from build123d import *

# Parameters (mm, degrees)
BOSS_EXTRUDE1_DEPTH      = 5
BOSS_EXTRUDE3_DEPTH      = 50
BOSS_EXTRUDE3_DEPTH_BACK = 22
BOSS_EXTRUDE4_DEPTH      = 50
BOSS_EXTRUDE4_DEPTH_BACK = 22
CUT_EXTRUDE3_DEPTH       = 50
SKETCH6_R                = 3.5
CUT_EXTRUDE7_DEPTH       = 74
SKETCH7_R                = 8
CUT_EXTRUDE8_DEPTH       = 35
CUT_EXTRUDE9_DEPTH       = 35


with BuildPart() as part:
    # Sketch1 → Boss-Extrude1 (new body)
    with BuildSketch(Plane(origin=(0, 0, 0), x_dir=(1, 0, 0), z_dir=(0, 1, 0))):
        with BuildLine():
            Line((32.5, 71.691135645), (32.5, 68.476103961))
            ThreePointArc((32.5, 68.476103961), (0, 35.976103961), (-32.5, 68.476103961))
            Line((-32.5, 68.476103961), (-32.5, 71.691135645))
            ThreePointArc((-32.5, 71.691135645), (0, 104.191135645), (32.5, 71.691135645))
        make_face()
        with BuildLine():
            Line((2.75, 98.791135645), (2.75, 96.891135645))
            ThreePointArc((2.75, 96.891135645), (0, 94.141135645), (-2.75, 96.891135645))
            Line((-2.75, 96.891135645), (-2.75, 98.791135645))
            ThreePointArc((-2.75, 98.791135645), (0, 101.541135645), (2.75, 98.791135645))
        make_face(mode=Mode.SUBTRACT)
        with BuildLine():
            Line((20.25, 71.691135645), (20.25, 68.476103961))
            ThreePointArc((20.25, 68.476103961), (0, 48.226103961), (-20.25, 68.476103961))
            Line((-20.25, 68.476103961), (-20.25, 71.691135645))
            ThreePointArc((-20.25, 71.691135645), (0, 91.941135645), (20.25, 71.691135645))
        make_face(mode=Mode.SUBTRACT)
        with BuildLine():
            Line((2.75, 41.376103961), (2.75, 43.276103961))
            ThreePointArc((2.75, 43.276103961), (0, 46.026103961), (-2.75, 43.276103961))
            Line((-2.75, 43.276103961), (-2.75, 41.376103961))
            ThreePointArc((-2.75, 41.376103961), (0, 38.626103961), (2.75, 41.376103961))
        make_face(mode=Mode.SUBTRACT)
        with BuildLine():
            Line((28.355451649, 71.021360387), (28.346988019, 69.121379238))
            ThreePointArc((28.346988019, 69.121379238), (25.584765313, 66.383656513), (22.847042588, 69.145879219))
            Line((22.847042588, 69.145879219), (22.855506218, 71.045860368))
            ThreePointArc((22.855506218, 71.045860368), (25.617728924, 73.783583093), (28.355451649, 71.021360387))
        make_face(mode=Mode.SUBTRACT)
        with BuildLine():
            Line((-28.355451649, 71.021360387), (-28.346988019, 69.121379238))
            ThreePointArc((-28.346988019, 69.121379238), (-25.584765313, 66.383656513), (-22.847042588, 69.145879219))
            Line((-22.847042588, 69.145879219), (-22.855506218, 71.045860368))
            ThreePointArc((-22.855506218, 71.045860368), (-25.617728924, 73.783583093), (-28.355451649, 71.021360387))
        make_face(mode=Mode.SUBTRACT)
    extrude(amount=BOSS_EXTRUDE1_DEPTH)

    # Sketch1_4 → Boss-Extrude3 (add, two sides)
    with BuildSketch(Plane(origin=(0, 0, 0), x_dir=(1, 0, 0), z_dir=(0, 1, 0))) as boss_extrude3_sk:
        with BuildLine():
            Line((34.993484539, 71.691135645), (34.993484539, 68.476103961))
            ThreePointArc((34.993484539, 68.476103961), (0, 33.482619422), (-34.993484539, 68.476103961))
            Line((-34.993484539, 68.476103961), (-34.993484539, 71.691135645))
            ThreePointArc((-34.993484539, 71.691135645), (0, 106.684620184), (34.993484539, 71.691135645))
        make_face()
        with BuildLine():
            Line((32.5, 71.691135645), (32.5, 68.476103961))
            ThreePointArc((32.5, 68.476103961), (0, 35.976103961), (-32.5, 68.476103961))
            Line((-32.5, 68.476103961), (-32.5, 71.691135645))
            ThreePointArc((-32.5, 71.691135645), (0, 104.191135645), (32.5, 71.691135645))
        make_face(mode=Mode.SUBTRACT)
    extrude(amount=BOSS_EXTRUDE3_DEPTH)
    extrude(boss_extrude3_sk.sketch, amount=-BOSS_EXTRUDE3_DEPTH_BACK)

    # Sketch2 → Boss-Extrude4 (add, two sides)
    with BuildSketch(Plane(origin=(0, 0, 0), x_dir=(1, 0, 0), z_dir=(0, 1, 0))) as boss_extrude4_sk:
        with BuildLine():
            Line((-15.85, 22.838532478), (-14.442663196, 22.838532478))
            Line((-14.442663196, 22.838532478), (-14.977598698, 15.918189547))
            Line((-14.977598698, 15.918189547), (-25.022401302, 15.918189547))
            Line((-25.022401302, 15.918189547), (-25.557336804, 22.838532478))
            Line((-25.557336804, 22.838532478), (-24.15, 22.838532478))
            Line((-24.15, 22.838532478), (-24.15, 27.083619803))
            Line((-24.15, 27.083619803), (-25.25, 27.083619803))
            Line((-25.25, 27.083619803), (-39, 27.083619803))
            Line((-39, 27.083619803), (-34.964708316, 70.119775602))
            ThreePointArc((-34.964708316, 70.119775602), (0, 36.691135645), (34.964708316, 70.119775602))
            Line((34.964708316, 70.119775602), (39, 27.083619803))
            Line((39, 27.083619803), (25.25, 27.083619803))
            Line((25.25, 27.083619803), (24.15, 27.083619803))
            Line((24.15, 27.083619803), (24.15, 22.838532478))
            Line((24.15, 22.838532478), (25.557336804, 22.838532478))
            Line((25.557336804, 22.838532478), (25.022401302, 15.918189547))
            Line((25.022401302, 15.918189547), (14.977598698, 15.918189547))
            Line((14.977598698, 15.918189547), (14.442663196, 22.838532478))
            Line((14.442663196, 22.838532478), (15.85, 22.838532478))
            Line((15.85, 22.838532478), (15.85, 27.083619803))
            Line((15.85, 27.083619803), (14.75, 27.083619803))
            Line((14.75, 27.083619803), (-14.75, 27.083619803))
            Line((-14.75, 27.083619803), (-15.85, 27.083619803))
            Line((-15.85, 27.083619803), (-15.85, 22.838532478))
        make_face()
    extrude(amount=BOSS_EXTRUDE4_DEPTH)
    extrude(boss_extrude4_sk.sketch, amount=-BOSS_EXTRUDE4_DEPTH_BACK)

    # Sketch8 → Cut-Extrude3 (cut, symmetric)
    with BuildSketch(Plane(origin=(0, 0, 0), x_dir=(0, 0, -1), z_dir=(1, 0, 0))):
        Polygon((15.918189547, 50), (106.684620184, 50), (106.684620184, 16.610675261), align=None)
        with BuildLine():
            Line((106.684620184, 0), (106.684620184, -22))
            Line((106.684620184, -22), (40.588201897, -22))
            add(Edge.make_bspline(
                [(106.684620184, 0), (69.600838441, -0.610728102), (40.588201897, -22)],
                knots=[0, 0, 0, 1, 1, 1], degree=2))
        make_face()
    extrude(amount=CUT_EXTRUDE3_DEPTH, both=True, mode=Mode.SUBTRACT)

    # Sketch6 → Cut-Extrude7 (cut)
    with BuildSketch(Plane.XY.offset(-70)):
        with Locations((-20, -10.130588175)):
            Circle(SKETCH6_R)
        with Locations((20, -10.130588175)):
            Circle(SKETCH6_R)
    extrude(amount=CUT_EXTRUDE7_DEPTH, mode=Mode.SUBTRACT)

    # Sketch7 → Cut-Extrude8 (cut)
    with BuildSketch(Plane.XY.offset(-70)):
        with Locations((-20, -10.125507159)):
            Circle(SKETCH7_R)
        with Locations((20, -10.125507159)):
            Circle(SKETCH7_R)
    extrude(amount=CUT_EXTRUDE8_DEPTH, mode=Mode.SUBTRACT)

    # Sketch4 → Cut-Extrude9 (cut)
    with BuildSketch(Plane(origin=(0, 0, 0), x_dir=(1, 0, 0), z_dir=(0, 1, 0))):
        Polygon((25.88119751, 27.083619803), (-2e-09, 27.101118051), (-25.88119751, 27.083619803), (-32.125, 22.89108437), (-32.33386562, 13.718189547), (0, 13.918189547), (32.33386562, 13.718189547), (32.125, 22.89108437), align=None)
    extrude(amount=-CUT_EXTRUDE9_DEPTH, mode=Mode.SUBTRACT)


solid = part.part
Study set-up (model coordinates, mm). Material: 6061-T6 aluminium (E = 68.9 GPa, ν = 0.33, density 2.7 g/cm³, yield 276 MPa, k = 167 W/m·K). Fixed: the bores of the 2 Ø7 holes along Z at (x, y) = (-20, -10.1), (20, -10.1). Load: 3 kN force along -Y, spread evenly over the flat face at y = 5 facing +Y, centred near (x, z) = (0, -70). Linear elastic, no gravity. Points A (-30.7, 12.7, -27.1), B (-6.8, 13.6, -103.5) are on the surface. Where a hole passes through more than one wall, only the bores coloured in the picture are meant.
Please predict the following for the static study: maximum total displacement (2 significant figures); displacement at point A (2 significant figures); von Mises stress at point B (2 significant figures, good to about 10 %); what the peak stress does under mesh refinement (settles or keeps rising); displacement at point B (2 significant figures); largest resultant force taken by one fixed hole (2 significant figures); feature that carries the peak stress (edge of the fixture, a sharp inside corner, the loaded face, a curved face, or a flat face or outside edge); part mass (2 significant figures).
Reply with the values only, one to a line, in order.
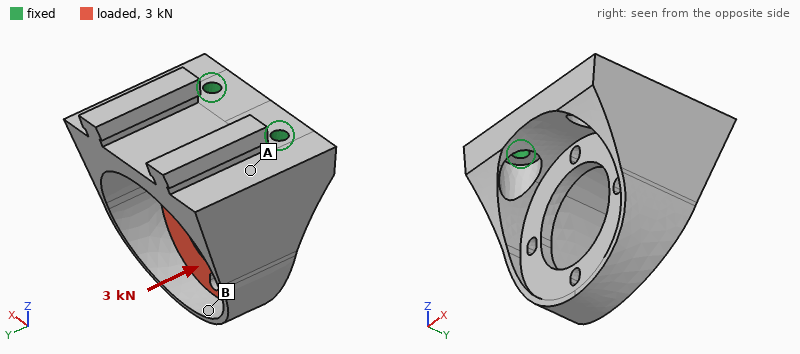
0.39 mm
0.065 mm
43 MPa
keeps rising
0.35 mm
1.5 kN
edge of the fixture
300 g
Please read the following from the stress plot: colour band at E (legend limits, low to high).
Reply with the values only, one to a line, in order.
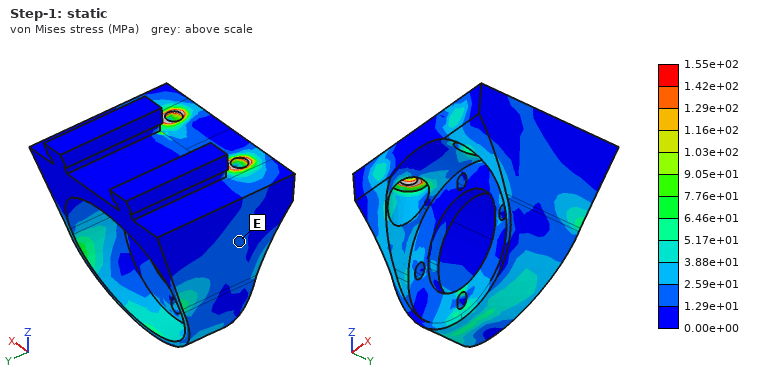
1.29e+01 to 2.59e+01 MPa
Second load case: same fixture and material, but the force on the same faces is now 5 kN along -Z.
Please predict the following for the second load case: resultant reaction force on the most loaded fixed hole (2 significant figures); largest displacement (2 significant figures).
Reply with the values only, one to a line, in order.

2.5 kN
0.17 mm
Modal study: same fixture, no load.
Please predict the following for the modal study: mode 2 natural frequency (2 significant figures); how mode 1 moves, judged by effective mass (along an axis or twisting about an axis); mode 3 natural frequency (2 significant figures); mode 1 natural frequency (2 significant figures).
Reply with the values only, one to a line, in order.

3000 Hz
along Z
4300 Hz
1600 Hz
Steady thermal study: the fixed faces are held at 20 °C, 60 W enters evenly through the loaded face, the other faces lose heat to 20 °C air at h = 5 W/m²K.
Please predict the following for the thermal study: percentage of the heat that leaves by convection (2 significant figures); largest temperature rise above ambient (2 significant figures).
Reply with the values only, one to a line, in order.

3.2 %
39 K
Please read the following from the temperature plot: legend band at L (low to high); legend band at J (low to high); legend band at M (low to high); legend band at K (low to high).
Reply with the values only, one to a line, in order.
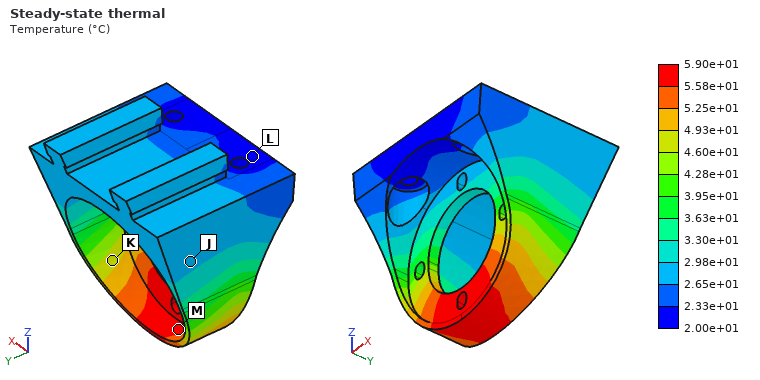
2.00e+01 to 2.33e+01 °C
2.65e+01 to 2.98e+01 °C
5.58e+01 to 5.90e+01 °C
4.60e+01 to 4.93e+01 °C
